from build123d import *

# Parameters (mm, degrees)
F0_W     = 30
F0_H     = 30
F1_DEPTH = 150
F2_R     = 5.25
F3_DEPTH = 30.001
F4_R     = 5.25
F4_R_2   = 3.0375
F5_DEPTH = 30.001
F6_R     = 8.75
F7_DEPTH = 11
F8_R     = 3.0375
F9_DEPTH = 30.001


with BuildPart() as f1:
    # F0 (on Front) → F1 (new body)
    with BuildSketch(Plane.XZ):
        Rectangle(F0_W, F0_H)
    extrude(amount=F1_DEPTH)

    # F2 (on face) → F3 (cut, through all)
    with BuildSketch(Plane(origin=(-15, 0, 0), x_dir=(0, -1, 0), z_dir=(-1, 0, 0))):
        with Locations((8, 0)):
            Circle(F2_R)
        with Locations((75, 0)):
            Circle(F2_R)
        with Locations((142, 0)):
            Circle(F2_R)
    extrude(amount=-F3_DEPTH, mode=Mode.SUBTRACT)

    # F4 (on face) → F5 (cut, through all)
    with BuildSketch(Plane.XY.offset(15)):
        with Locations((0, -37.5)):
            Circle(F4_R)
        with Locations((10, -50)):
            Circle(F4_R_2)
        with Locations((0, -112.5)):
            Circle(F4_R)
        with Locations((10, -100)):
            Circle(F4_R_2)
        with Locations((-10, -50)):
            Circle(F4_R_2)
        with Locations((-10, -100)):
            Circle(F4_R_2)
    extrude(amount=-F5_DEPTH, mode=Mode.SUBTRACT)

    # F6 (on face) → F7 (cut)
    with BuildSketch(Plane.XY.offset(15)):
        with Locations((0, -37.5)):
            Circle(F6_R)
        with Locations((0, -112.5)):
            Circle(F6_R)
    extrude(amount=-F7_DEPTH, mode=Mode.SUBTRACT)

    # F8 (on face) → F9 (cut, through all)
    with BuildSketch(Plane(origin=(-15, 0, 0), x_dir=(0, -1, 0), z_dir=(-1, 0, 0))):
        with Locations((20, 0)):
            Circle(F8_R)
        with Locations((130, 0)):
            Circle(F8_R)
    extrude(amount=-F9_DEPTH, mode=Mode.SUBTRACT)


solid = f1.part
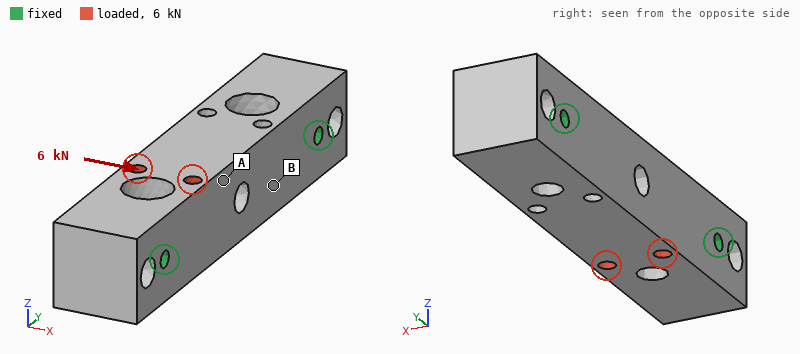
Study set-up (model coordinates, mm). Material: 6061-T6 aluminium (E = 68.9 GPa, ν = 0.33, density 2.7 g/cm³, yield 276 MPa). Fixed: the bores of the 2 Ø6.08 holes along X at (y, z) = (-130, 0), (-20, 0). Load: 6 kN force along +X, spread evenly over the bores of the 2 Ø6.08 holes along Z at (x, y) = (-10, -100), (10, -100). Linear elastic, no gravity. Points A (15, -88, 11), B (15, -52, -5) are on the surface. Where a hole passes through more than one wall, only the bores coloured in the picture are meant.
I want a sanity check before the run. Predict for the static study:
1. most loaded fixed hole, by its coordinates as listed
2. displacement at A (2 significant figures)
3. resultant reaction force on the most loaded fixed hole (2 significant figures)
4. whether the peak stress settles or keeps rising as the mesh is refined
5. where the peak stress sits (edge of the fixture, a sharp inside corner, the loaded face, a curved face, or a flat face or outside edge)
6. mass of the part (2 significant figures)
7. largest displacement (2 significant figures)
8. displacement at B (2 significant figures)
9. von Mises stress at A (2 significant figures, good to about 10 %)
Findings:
(-130, 0)
22 µm
4.7 kN
keeps rising
edge of the fixture
310 g
25 µm
11 µm
10 MPa
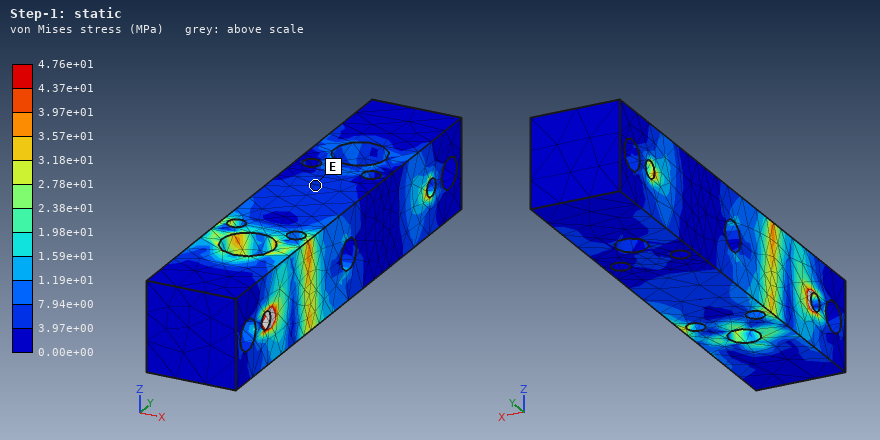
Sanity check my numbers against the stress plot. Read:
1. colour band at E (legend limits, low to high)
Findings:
3.97e+00 to 7.94e+00 MPa
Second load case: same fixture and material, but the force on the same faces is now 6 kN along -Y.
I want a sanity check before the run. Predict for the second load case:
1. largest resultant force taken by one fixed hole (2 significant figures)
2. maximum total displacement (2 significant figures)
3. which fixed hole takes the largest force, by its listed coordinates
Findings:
4.2 kN
4.0 µm
(-130, 0)
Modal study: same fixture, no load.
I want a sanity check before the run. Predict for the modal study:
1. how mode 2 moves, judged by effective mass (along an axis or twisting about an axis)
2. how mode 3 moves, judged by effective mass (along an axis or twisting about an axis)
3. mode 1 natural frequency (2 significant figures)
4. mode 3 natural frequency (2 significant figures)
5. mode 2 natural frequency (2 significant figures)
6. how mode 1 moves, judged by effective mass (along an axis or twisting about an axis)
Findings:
along X
twisting about Y
6300 Hz
11 kHz
7300 Hz
along Z
